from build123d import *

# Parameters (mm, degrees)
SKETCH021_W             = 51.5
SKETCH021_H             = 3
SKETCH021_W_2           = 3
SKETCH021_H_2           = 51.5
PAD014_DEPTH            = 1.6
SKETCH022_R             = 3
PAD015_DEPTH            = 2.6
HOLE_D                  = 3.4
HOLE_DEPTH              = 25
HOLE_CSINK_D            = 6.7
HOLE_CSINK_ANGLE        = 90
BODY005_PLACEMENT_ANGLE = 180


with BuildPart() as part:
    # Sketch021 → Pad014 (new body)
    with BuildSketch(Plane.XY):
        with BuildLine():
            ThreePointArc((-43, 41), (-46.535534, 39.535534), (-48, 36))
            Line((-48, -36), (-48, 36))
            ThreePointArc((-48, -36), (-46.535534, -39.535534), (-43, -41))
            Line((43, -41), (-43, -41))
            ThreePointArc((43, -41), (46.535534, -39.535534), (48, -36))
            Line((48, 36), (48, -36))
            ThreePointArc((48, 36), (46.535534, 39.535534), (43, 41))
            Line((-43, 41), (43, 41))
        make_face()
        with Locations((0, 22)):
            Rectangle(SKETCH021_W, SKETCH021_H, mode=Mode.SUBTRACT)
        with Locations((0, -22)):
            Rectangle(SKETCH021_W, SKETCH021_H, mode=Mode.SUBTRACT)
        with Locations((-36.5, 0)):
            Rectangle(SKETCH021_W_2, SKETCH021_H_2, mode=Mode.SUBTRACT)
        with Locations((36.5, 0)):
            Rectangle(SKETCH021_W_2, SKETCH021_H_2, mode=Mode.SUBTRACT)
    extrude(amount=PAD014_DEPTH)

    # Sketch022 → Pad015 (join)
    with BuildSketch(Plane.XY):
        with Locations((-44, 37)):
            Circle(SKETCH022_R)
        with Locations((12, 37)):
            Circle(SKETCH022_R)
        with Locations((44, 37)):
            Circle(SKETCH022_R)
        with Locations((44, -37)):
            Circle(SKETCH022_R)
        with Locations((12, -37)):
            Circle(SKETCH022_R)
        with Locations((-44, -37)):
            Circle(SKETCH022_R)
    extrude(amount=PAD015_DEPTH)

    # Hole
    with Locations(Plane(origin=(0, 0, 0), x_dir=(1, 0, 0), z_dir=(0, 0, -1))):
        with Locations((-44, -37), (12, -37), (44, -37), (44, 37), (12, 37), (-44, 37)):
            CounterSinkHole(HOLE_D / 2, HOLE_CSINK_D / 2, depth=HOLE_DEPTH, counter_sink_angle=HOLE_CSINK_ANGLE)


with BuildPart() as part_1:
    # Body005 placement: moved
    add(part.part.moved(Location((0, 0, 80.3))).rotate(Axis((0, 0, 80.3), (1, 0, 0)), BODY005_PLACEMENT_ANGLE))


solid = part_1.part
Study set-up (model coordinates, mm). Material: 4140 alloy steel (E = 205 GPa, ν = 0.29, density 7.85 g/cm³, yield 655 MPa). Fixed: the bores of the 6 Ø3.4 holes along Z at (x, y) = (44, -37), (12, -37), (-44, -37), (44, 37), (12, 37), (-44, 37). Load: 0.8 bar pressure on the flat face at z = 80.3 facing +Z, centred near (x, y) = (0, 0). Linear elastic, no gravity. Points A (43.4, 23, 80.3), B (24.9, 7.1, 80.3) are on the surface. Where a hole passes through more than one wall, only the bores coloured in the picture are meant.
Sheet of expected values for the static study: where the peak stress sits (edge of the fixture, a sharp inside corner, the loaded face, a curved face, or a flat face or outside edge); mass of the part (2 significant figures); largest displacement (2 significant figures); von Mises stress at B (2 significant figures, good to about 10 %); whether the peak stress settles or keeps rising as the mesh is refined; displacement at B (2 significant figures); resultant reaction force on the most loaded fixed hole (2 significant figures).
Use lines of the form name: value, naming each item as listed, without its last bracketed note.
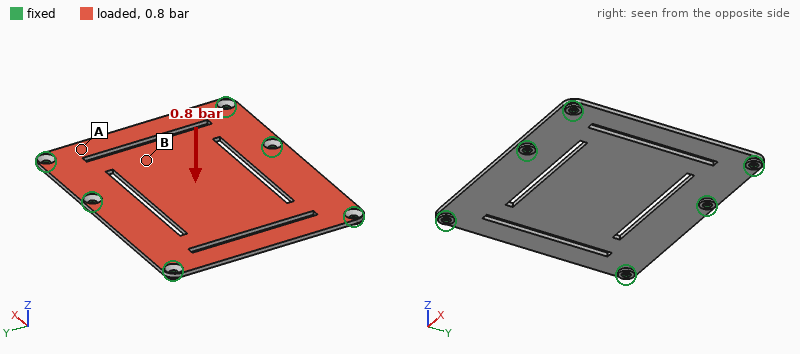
where the peak stress sits: edge of the fixture
mass of the part: 90 g
largest displacement: 0.25 mm
von Mises stress at B: 56 MPa
whether the peak stress settles or keeps rising as the mesh is refined: keeps rising
displacement at B: 0.16 mm
resultant reaction force on the most loaded fixed hole: 260 N
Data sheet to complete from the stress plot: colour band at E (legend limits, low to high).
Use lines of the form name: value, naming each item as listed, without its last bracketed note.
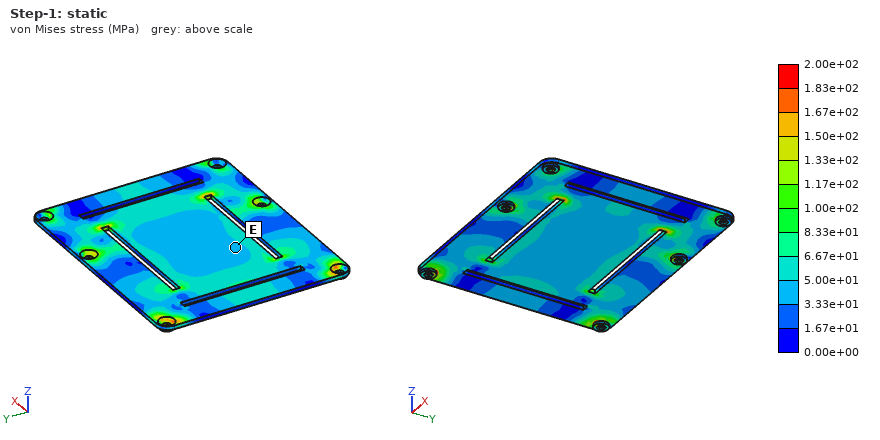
colour band at E: 3.33e+01 to 5.00e+01 MPa
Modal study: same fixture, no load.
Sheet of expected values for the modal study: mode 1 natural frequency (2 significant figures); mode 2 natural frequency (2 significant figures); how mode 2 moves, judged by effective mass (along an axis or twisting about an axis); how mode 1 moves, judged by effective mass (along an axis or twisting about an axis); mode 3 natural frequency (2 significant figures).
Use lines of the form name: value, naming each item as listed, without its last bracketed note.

mode 1 natural frequency: 950 Hz
mode 2 natural frequency: 1500 Hz
how mode 2 moves, judged by effective mass: twisting about Y
how mode 1 moves, judged by effective mass: along Z
mode 3 natural frequency: 1800 Hz
